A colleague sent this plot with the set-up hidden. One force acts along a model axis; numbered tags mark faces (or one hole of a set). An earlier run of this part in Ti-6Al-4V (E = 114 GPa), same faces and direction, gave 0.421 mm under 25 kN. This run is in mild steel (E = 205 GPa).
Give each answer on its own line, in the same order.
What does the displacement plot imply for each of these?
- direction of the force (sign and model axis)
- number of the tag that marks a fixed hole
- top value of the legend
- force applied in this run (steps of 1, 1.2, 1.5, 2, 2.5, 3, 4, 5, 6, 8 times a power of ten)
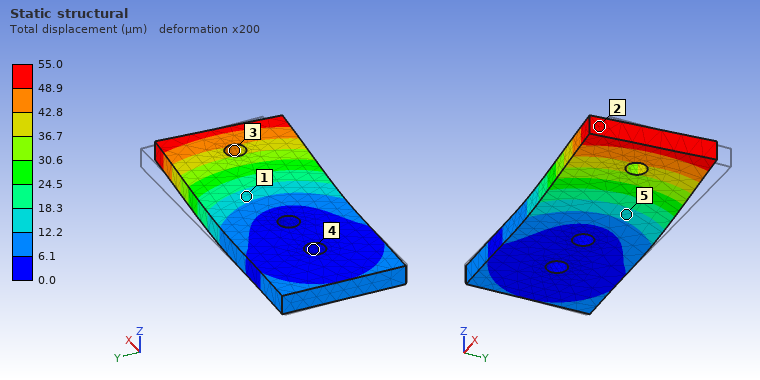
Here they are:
-Y
4
55.0 µm
6 kN
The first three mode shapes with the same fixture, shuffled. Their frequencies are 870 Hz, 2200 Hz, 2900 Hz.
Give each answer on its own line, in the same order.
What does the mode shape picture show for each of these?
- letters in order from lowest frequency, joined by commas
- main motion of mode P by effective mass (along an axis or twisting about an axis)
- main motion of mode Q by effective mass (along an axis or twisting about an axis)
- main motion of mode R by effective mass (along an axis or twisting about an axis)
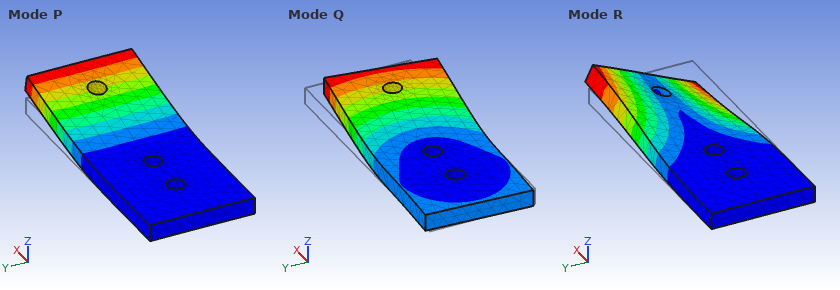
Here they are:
P, R, Q
along Z
along Y
twisting about X
